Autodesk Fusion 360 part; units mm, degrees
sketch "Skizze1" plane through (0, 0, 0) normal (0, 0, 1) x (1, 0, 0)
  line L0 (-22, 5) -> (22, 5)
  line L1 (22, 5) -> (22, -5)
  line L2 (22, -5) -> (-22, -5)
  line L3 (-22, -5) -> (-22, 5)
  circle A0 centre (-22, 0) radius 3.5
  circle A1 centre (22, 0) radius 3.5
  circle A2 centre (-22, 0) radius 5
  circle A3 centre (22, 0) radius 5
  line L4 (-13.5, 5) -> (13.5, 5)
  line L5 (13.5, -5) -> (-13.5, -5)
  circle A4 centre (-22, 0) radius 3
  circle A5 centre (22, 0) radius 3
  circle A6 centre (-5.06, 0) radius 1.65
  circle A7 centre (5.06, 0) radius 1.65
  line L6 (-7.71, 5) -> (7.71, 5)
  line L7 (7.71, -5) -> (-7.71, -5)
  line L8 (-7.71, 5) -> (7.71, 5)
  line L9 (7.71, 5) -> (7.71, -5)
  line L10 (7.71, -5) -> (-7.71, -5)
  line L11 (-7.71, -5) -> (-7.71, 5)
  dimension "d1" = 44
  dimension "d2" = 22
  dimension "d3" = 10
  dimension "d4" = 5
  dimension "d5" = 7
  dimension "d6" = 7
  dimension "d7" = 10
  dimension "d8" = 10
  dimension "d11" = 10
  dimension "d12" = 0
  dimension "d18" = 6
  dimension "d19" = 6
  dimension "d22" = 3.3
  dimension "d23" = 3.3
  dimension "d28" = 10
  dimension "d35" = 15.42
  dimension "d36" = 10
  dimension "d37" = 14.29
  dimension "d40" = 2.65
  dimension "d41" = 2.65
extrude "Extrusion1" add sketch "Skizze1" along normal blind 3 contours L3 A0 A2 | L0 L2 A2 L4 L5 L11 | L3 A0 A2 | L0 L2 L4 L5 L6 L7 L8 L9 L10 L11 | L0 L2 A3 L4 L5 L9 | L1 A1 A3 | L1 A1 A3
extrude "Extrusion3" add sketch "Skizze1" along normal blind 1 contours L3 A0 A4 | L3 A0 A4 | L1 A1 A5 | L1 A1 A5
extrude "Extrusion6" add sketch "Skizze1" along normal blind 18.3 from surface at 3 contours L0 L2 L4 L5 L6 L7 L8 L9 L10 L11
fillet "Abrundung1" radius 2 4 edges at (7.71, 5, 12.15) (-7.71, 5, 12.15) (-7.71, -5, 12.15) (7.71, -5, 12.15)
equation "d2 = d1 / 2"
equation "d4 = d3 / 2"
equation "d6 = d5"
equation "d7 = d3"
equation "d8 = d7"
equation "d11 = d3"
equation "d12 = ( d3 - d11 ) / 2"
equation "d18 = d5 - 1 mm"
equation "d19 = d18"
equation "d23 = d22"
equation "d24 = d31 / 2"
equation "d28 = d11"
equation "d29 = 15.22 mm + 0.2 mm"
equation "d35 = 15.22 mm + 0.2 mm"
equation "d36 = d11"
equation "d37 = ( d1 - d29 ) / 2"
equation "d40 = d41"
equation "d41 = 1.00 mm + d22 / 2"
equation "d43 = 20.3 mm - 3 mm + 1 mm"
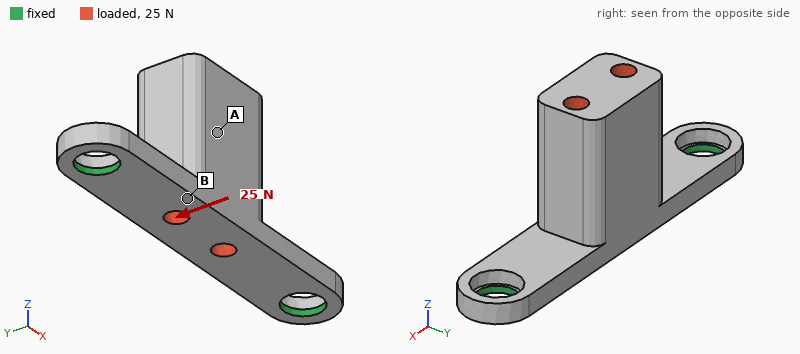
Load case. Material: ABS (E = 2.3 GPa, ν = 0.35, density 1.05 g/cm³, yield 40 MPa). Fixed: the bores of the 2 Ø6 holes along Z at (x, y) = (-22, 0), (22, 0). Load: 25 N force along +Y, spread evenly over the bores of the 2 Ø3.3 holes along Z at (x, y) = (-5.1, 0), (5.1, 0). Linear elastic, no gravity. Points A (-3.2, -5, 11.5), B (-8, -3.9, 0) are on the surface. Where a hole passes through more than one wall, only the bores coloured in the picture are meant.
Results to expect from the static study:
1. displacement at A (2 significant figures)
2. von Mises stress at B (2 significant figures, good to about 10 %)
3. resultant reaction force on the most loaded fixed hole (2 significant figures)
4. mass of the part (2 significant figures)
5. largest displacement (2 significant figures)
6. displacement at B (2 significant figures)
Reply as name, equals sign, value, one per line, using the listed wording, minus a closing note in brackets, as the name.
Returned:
displacement at A = 0.34 mm
von Mises stress at B = 4.5 MPa
resultant reaction force on the most loaded fixed hole = 13 N
mass of the part = 3.9 g
largest displacement = 0.60 mm
displacement at B = 0.10 mm
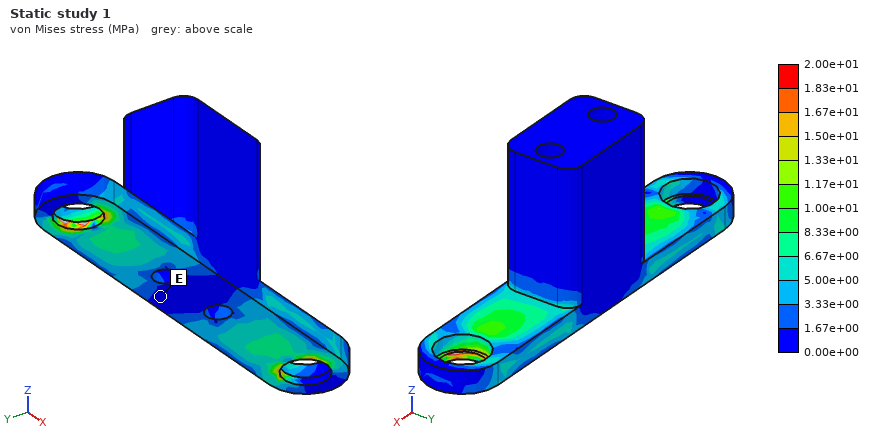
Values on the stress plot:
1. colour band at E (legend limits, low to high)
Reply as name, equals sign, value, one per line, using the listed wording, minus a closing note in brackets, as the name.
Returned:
colour band at E = 0.00e+00 to 1.67e+00 MPa
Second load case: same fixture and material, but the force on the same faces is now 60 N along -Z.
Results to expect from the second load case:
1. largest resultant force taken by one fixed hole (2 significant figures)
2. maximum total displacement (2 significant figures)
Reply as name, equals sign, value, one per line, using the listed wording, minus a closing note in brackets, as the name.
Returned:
largest resultant force taken by one fixed hole = 63 N
maximum total displacement = 0.21 mm
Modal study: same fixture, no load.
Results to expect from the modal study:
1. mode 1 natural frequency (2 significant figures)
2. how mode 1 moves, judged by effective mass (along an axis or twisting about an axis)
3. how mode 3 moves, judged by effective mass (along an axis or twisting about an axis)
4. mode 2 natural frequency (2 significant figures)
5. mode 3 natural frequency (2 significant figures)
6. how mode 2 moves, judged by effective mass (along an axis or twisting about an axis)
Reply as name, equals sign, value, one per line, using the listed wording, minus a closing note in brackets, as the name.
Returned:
mode 1 natural frequency = 710 Hz
how mode 1 moves, judged by effective mass = along Y
how mode 3 moves, judged by effective mass = along X
mode 2 natural frequency = 1500 Hz
mode 3 natural frequency = 1800 Hz
how mode 2 moves, judged by effective mass = along Z
